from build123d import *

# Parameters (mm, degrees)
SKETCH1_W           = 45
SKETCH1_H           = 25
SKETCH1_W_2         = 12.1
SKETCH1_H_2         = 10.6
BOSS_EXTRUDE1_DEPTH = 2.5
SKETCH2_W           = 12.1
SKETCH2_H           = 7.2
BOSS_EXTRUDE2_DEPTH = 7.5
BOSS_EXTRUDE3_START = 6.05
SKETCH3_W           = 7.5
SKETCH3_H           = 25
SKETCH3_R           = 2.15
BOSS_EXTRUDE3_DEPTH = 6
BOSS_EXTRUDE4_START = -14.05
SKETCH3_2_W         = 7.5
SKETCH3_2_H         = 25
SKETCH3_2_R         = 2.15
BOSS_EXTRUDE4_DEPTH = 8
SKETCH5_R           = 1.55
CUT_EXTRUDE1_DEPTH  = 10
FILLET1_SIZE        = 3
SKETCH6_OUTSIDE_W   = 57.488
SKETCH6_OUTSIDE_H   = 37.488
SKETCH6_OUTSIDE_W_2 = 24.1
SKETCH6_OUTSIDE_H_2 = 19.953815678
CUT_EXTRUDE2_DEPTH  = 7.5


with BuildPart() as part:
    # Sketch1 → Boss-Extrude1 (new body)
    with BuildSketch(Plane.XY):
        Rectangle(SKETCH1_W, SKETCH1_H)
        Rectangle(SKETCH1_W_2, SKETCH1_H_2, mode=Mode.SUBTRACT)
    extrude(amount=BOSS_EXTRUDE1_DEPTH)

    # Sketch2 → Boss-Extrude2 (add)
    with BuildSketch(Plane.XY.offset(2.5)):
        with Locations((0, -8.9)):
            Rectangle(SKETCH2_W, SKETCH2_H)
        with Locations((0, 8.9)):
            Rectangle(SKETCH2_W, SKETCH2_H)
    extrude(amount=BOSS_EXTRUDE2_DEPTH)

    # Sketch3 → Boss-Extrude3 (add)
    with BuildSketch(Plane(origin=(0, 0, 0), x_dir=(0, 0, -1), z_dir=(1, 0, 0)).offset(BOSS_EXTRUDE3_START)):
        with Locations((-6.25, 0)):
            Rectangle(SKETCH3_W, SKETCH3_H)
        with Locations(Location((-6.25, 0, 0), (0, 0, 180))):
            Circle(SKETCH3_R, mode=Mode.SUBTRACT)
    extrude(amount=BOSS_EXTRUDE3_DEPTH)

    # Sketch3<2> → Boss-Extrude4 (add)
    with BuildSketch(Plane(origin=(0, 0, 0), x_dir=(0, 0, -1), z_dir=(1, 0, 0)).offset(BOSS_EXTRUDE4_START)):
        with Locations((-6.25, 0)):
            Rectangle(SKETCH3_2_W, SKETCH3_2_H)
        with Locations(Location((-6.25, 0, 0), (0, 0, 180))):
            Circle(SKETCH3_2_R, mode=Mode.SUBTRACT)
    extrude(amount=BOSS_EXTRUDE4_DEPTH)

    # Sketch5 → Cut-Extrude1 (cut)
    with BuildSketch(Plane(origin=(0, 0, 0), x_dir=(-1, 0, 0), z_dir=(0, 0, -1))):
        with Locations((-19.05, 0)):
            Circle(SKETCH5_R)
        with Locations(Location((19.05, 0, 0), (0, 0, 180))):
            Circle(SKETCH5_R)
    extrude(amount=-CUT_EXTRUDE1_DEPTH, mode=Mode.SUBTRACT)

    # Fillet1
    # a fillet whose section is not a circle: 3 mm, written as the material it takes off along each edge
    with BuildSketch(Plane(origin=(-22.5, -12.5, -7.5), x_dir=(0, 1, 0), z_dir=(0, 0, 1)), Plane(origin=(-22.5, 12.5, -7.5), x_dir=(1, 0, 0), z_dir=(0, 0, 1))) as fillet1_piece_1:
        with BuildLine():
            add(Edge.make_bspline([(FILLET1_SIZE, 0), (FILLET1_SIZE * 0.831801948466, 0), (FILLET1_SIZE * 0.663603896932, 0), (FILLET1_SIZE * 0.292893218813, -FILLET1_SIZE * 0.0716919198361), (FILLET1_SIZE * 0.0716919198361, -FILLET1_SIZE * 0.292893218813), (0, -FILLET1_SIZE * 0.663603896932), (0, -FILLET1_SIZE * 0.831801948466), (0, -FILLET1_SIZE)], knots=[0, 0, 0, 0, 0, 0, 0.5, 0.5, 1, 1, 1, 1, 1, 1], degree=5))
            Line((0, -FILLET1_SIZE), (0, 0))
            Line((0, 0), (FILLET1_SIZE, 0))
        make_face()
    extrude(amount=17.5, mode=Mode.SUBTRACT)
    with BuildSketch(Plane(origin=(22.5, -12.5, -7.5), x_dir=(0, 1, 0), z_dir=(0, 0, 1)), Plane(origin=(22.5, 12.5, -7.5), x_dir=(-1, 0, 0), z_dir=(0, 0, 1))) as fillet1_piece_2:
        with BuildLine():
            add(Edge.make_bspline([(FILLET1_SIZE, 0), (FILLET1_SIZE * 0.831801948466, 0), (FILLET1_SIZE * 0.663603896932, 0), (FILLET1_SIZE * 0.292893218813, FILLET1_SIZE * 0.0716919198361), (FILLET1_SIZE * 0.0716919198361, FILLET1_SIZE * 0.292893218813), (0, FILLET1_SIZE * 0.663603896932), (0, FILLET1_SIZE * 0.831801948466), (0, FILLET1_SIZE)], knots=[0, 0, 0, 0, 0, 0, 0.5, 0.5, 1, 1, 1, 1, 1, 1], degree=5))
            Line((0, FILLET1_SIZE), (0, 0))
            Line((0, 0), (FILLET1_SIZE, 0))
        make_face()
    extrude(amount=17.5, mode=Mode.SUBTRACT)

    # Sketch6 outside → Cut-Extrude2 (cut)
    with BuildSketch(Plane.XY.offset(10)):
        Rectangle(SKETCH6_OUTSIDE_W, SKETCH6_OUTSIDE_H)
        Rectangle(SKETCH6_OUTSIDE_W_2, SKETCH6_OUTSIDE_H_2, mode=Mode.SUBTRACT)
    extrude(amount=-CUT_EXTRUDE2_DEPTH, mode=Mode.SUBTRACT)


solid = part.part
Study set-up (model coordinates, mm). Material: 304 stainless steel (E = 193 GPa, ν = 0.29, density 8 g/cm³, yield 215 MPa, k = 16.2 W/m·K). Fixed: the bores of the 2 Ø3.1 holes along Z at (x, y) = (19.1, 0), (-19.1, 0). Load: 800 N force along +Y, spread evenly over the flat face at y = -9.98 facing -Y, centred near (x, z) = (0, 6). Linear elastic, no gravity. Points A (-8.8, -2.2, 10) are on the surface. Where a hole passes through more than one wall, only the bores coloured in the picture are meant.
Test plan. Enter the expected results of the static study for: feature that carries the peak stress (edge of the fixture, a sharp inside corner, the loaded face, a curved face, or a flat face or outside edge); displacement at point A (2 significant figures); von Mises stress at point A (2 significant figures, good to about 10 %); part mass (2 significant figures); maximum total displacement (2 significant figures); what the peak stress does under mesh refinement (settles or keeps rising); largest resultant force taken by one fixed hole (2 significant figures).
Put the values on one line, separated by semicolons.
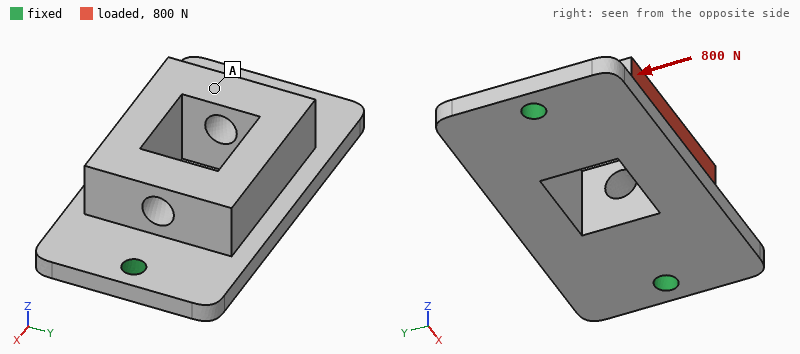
edge of the fixture; 17 µm; 20 MPa; 39 g; 26 µm; keeps rising; 400 N
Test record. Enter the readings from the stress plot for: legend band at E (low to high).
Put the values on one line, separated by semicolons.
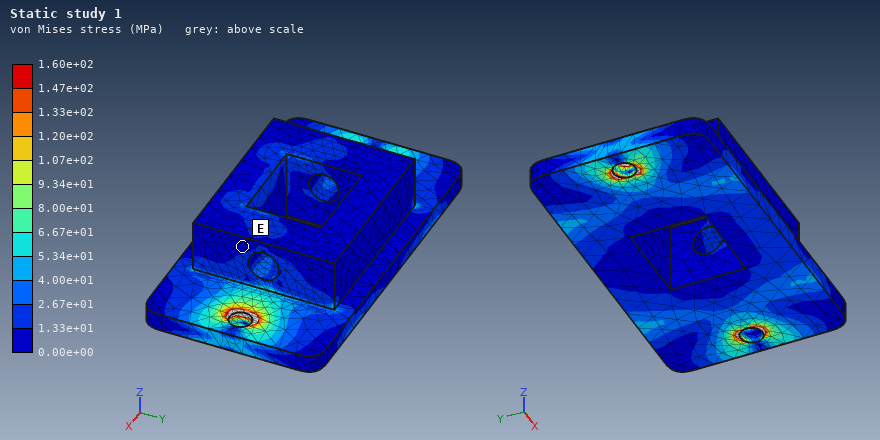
0.00e+00 to 1.33e+01 MPa
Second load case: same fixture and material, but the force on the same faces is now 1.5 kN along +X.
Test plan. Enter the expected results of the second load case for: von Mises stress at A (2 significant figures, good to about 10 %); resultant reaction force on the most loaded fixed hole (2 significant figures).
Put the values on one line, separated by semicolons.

15 MPa; 870 N
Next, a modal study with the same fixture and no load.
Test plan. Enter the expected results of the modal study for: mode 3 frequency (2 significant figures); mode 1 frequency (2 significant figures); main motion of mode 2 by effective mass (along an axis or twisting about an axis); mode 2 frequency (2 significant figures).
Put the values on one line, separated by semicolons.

15 kHz; 5000 Hz; along Z; 9200 Hz
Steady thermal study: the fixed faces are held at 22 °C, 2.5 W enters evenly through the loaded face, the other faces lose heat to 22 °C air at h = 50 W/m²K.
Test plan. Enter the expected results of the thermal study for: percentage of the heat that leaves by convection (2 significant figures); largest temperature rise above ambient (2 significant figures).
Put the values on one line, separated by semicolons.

50 %; 19 K
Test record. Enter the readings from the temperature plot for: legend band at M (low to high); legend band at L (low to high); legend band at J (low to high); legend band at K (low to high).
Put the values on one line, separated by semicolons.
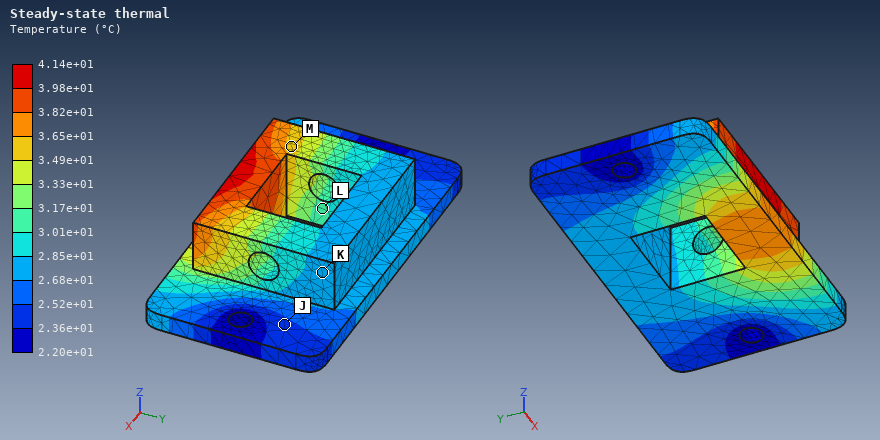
3.49e+01 to 3.65e+01 °C; 3.01e+01 to 3.17e+01 °C; 2.36e+01 to 2.52e+01 °C; 2.68e+01 to 2.85e+01 °C
